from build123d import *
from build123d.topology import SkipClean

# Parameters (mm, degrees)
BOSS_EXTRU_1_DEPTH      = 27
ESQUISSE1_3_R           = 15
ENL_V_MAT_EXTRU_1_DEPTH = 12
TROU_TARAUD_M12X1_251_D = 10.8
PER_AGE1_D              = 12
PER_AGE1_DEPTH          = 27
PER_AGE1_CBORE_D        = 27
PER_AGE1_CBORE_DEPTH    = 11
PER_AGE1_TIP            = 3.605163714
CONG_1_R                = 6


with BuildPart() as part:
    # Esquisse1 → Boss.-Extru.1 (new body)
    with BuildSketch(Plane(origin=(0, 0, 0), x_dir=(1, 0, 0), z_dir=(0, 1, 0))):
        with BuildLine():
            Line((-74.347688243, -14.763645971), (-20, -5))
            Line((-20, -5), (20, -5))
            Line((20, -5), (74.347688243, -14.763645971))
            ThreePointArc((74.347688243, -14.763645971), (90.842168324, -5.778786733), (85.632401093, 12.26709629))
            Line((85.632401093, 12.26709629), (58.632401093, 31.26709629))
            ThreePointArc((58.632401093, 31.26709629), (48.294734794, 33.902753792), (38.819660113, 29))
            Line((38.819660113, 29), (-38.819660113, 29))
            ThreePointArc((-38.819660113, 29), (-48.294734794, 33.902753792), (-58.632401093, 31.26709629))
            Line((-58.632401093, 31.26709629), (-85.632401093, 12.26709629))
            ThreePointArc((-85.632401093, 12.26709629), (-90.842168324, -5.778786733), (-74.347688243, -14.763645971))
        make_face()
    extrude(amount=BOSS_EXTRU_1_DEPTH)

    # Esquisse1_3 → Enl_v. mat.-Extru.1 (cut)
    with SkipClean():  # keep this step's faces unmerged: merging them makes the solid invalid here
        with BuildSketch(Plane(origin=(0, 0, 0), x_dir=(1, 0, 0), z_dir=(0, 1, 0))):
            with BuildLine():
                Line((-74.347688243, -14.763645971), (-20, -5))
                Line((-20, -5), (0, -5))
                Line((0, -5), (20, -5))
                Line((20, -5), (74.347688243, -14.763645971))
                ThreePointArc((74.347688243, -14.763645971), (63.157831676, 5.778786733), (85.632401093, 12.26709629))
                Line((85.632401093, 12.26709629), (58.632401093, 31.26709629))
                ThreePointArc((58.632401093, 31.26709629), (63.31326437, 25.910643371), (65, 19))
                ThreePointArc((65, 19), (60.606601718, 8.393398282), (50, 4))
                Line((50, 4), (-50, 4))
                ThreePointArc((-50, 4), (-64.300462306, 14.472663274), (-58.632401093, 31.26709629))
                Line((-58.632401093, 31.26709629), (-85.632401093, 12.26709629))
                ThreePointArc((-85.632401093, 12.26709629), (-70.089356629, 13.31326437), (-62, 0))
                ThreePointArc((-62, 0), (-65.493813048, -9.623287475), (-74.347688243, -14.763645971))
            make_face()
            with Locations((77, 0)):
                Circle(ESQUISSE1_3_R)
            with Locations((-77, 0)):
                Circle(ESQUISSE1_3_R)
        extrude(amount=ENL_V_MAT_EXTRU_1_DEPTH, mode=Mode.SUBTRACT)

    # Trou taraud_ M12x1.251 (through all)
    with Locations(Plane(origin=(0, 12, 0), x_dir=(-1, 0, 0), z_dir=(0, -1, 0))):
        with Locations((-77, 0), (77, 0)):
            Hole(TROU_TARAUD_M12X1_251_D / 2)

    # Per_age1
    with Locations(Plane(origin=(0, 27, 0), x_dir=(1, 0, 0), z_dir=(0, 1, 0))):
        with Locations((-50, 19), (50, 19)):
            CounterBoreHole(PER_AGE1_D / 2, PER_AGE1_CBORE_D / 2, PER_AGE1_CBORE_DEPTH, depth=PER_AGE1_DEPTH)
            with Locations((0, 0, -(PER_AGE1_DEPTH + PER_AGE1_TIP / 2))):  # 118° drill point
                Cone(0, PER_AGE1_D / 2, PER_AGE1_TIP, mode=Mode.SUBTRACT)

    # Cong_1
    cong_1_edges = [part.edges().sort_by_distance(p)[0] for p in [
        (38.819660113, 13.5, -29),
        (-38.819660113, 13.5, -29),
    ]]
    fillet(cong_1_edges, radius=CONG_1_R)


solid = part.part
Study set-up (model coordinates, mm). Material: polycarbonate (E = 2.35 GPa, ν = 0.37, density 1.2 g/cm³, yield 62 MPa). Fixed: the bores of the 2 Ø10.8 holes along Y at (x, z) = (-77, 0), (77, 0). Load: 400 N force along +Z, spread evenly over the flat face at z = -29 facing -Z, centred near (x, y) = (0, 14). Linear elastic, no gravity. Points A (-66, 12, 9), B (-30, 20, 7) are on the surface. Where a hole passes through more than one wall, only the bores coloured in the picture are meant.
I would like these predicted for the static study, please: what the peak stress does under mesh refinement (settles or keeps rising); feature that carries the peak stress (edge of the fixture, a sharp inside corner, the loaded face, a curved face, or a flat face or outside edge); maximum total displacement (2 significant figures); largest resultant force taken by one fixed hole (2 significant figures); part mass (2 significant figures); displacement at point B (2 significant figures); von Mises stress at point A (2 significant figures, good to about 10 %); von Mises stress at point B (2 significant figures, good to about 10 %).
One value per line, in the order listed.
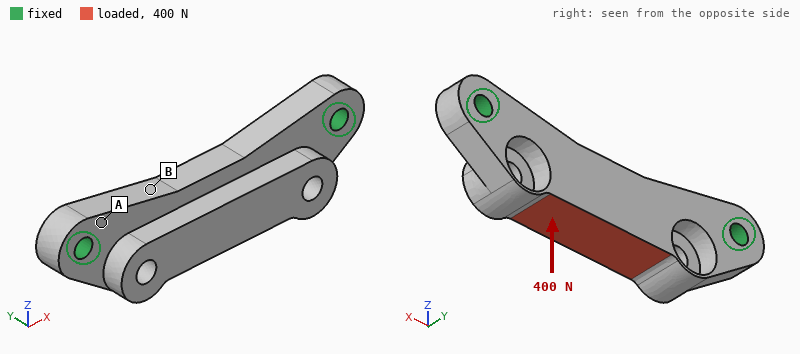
keeps rising
edge of the fixture
0.13 mm
270 N
140 g
0.074 mm
1.6 MPa
0.58 MPa
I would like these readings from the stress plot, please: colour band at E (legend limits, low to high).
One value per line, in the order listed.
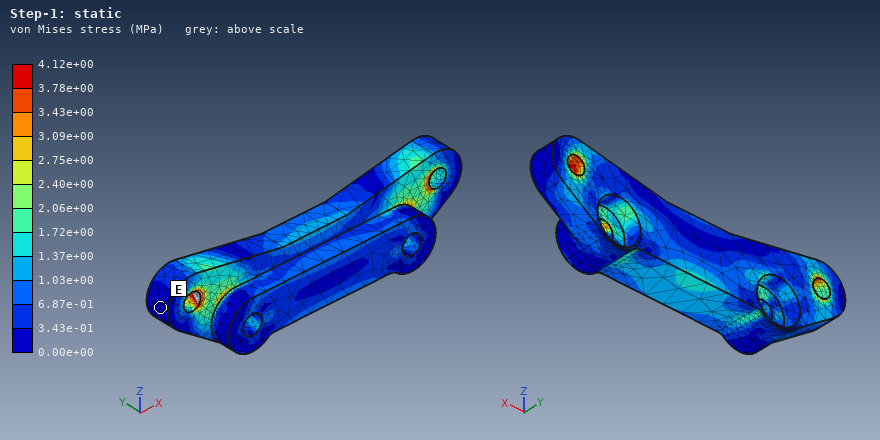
0.00e+00 to 3.43e-01 MPa
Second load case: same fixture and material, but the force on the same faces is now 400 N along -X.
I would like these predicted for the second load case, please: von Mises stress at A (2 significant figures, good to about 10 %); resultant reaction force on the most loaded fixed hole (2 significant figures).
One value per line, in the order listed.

0.54 MPa
220 N
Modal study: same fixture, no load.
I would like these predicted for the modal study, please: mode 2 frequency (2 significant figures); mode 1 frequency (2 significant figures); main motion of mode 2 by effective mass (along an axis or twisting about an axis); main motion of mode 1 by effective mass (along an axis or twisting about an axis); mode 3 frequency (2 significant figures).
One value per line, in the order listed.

1300 Hz
820 Hz
along Z
along Y
1600 Hz
